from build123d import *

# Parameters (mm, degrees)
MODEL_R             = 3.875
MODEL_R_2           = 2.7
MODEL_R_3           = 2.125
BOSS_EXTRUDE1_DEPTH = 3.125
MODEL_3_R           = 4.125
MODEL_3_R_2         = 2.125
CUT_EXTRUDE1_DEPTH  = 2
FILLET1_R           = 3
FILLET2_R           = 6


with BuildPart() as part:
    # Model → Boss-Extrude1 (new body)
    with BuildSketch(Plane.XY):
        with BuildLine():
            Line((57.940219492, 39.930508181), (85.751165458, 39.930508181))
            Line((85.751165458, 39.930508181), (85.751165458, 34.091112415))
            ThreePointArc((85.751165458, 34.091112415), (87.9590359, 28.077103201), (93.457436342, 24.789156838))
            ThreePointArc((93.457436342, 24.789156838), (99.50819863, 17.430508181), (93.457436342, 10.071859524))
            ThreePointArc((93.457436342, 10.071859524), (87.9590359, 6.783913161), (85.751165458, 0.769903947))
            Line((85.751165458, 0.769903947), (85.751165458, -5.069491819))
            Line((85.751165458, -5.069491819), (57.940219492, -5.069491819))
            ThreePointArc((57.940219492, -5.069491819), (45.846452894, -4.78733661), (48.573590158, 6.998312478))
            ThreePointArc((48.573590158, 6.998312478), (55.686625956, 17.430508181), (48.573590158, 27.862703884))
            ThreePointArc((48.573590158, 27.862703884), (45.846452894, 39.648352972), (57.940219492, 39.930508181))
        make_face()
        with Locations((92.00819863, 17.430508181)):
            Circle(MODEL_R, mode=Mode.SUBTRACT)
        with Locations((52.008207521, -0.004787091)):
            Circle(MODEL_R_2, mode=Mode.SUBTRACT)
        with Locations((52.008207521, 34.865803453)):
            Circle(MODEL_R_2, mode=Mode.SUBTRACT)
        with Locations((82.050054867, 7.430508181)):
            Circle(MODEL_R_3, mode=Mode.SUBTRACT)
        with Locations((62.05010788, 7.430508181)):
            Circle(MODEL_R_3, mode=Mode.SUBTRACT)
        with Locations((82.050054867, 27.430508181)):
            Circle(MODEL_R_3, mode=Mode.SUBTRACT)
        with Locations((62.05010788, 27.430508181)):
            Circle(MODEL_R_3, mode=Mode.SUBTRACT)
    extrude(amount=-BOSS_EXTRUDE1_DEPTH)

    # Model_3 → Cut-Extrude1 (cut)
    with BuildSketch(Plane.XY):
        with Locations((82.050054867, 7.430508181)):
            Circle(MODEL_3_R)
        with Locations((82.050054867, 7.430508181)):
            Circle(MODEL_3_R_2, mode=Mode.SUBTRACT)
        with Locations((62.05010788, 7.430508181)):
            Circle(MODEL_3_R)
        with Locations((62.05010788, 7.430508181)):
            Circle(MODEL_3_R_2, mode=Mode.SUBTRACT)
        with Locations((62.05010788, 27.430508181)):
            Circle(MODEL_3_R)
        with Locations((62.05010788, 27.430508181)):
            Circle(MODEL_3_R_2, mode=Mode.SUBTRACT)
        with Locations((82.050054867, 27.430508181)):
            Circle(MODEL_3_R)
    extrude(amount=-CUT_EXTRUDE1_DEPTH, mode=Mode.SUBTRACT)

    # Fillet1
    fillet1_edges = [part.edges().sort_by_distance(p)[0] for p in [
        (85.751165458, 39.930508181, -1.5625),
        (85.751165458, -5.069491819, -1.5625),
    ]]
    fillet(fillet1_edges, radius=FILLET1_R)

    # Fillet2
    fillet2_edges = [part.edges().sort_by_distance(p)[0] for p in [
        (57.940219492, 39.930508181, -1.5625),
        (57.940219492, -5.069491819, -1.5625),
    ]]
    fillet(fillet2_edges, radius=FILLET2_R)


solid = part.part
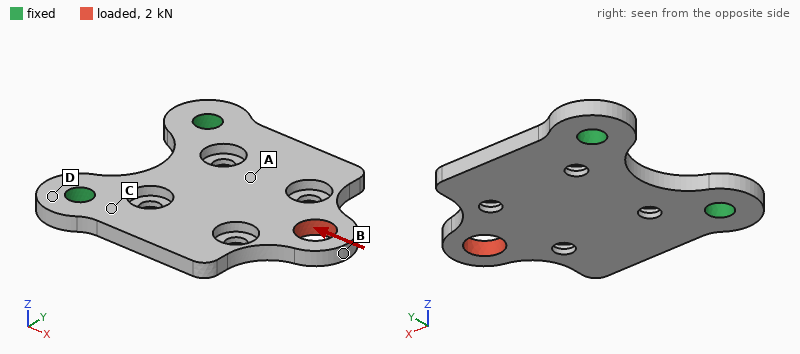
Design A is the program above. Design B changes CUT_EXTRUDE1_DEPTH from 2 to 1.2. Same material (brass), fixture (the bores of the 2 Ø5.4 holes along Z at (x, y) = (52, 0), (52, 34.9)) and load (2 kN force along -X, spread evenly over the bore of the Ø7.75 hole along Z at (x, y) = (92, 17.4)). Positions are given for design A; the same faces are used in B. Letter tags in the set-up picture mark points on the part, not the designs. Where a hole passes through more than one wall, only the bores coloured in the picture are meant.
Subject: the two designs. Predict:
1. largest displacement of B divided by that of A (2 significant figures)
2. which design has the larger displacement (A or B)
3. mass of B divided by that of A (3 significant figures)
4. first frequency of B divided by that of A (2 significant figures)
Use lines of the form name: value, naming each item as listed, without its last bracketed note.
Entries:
largest displacement of B divided by that of A: 0.84
which design has the larger displacement: A
mass of B divided by that of A: 1.02
first frequency of B divided by that of A: 0.99
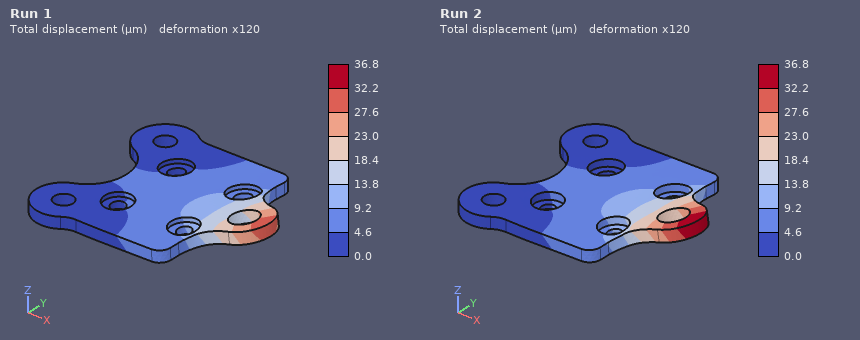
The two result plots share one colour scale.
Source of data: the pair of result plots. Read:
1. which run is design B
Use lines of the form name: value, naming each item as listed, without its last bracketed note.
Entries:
which run is design B: Run 1
